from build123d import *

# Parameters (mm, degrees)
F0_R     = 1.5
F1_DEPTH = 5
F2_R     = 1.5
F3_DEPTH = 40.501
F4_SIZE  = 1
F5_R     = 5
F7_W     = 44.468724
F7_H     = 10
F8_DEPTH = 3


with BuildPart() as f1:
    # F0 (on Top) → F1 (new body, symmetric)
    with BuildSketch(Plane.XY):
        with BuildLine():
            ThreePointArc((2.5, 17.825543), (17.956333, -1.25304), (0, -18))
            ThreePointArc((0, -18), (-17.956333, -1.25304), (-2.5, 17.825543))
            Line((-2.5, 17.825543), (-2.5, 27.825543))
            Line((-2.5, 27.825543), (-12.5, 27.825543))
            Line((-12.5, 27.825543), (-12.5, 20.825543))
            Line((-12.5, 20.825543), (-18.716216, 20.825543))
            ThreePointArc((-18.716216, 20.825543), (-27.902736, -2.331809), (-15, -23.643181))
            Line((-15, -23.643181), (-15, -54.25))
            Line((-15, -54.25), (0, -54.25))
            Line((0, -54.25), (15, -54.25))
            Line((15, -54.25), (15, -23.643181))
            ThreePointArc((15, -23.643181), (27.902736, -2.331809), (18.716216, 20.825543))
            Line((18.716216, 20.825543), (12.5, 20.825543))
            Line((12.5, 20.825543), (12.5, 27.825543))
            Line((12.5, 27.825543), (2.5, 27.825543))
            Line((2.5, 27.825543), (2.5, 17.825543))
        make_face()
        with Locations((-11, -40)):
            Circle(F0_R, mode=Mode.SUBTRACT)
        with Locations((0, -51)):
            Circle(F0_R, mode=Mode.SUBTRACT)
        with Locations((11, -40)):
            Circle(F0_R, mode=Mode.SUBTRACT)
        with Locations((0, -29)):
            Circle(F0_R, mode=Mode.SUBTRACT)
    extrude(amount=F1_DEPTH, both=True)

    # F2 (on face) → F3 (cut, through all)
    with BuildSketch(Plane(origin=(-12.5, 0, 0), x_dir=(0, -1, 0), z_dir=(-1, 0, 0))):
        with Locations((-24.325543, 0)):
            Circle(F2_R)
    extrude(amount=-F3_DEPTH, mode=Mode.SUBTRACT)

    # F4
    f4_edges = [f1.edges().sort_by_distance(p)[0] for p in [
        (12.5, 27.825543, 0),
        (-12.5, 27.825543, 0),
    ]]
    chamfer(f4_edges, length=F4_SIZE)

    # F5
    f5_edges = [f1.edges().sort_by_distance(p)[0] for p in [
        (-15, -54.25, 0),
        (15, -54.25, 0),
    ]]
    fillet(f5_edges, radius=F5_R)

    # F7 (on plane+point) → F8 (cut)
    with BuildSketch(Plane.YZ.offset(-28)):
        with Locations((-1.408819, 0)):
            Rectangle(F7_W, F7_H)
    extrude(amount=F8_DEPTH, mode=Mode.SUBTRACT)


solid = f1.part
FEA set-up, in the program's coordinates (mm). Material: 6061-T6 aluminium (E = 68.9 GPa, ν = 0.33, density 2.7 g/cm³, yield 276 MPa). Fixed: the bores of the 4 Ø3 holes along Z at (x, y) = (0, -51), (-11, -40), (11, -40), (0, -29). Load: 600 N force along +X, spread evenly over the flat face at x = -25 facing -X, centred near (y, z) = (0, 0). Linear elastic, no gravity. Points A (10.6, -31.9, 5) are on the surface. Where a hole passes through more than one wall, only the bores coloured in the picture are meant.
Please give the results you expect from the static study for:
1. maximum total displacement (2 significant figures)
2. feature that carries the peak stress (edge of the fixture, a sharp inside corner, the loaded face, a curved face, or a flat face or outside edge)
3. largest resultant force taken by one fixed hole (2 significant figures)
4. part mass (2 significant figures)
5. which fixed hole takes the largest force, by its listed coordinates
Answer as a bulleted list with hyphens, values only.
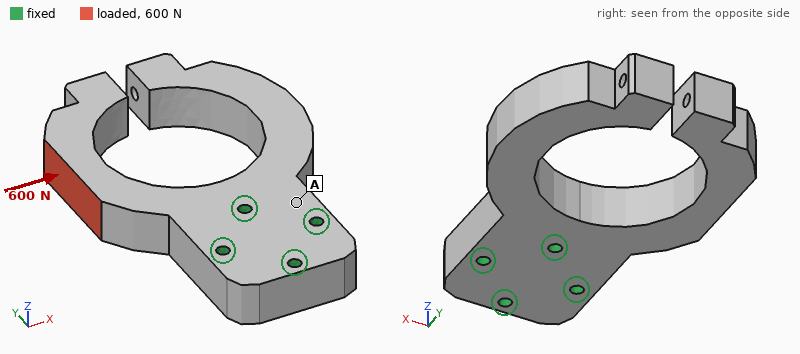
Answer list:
- 0.22 mm
- a curved face
- 1000 N
- 57 g
- (0, -29)
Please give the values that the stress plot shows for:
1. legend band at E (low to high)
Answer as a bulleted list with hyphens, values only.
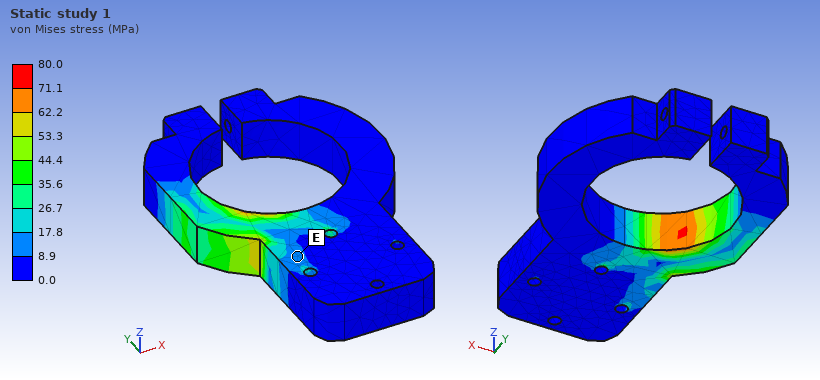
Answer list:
- 8.9 to 17.8 MPa
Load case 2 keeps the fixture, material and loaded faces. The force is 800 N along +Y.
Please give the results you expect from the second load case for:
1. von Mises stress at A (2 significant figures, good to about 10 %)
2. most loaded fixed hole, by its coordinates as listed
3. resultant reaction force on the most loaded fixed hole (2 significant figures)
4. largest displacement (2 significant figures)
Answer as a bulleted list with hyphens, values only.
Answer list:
- 3.8 MPa
- (-11, -40)
- 1.0 kN
- 0.17 mm
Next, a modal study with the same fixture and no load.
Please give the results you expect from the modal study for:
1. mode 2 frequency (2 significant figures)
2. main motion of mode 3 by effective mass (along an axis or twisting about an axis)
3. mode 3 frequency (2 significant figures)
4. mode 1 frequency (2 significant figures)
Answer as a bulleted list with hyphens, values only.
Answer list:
- 2000 Hz
- along X
- 2200 Hz
- 2000 Hz
